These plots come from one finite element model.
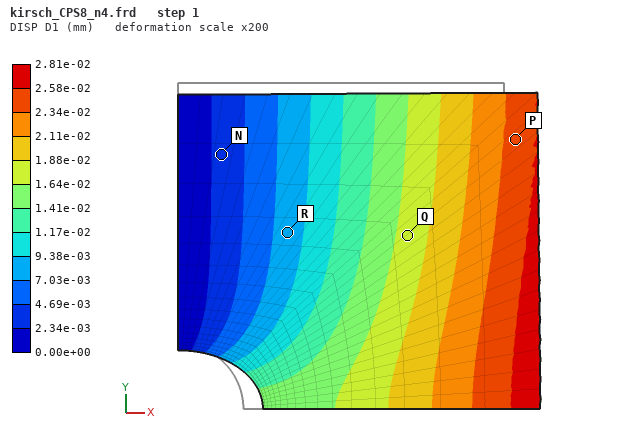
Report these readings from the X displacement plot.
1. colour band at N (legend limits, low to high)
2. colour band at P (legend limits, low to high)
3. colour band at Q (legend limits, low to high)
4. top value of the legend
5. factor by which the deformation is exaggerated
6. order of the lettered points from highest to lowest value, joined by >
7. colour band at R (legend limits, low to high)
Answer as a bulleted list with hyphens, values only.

- 2.34e-03 to 4.69e-03 mm
- 2.34e-02 to 2.58e-02 mm
- 1.64e-02 to 1.88e-02 mm
- 2.81e-02 mm
- 200
- P > Q > R > N
- 7.03e-03 to 9.38e-03 mm
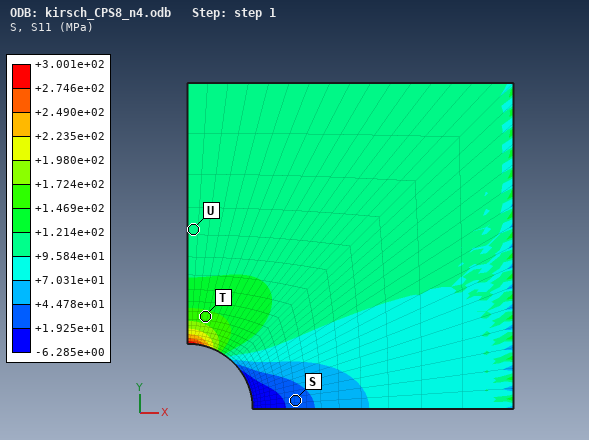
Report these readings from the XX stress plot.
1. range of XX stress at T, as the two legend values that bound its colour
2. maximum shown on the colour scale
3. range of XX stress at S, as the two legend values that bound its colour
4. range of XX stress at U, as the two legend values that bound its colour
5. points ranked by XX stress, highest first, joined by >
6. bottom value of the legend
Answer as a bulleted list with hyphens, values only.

- +1.469e+02 to +1.724e+02 MPa
- +3.001e+02 MPa
- +1.925e+01 to +4.478e+01 MPa
- +9.584e+01 to +1.214e+02 MPa
- T > U > S
- -6.285e+00 MPa
